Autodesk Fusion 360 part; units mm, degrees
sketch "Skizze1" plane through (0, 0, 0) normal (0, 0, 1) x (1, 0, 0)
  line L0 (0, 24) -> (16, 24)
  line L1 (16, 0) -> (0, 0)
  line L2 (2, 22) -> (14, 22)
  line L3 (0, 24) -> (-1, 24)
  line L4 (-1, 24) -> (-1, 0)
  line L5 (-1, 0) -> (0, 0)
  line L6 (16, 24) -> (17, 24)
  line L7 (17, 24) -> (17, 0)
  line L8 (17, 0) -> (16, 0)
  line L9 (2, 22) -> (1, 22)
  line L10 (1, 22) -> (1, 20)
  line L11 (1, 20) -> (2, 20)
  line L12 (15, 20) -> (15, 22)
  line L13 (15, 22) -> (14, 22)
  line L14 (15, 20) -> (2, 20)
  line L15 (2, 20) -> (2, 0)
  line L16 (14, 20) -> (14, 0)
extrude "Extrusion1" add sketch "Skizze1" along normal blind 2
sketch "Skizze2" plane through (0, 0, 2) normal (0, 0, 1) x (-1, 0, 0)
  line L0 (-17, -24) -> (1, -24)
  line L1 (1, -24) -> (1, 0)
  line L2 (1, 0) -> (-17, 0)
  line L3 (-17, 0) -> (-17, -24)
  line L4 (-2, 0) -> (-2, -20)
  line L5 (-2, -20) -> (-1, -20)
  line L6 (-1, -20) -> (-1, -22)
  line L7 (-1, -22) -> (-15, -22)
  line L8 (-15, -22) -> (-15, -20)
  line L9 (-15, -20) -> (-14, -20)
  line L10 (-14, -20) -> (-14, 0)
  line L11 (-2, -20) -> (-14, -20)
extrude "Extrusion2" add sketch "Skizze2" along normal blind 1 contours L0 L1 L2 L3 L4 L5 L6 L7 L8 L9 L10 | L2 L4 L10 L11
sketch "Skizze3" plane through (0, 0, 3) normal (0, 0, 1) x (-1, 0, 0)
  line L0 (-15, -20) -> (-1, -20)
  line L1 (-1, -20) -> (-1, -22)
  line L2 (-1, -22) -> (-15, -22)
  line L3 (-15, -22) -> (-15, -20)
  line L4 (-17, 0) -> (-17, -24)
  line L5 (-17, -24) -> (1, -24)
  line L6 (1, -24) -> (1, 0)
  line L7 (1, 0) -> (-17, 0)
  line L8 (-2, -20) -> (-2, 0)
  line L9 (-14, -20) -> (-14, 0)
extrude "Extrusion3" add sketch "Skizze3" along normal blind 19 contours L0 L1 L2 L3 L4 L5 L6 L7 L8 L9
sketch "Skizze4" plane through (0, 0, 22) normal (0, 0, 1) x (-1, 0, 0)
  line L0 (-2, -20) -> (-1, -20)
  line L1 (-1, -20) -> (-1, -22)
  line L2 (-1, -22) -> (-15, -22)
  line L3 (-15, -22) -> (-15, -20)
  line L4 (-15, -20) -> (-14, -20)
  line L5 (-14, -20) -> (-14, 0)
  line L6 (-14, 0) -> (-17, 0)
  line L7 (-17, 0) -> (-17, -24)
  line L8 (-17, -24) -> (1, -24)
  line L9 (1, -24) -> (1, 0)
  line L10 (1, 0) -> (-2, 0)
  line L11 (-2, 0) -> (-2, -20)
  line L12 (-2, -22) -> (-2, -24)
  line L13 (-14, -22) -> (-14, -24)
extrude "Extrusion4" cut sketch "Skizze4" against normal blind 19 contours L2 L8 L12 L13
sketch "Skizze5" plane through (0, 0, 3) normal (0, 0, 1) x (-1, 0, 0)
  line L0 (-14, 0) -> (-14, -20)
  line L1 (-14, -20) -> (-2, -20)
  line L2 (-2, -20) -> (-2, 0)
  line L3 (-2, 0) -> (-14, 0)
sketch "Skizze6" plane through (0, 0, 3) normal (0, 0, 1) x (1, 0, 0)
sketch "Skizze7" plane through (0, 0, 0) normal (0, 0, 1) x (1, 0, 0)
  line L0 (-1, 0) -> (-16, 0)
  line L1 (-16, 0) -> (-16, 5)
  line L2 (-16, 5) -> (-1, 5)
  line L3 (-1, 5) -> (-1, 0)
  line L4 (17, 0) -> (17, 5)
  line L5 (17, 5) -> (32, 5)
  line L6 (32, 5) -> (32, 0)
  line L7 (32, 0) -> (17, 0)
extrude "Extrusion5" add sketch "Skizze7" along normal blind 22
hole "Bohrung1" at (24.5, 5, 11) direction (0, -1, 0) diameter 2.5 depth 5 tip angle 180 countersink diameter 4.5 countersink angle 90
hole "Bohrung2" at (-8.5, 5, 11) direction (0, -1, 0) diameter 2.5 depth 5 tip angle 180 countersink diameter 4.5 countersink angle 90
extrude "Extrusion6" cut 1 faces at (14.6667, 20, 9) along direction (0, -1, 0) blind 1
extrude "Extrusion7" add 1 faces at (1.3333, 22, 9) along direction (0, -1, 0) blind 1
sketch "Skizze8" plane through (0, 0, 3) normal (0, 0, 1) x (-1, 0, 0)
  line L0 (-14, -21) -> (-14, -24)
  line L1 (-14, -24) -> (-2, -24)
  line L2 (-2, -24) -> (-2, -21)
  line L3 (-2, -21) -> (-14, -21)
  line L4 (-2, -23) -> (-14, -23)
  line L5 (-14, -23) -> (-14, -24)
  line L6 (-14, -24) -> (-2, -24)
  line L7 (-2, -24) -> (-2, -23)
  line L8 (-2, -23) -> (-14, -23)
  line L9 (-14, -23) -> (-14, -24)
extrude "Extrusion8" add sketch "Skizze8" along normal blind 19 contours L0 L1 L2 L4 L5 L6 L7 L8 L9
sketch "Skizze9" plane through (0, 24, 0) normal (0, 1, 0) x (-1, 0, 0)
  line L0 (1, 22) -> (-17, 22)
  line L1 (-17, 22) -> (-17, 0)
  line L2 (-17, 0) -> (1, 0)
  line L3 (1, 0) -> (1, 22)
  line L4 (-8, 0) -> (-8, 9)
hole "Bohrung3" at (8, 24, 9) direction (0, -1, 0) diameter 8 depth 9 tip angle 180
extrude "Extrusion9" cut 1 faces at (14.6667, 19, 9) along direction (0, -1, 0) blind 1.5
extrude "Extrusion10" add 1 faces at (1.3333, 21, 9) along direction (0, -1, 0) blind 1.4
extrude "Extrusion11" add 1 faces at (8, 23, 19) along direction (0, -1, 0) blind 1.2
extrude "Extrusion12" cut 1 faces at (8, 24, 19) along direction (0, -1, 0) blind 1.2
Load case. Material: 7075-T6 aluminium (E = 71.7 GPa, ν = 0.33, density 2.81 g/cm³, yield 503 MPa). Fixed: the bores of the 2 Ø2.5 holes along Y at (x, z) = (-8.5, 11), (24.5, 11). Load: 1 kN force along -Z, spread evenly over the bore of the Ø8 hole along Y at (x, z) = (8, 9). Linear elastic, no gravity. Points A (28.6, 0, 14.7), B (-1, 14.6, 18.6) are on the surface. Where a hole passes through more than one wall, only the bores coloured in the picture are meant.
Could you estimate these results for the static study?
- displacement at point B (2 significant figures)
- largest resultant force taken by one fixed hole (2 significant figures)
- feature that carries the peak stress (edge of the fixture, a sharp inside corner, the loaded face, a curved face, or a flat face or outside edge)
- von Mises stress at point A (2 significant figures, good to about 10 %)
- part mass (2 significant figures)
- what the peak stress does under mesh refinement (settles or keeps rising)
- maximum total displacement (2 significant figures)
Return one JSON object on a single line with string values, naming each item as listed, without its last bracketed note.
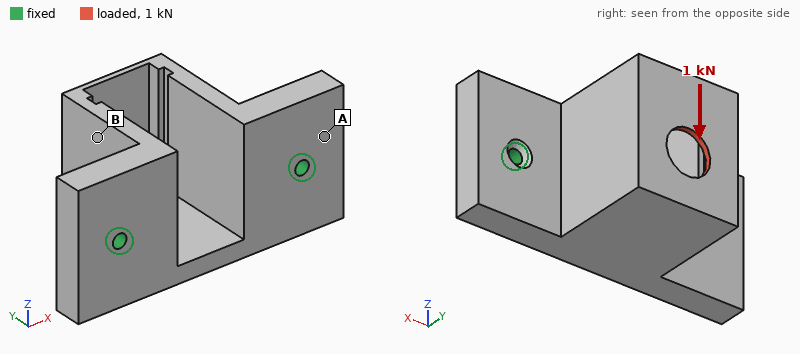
{"displacement at point B": "0.100 mm", "largest resultant force taken by one fixed hole": "620 N", "feature that carries the peak stress": "edge of the fixture", "von Mises stress at point A": "49 MPa", "part mass": "20 g", "what the peak stress does under mesh refinement": "keeps rising", "maximum total displacement": "0.16 mm"}
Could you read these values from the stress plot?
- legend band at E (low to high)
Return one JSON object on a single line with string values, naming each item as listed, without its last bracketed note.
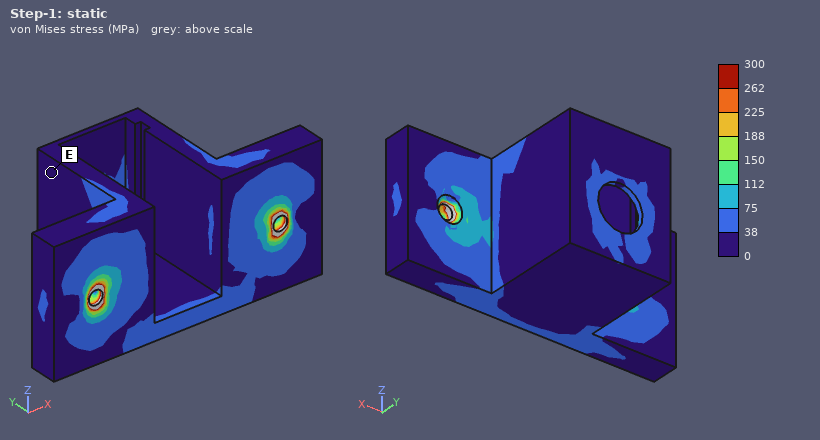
{"legend band at E": "0 to 38 MPa"}
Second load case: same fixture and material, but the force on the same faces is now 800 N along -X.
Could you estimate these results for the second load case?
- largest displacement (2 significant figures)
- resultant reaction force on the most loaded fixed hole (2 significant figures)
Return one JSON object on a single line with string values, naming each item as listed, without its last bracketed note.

{"largest displacement": "0.14 mm", "resultant reaction force on the most loaded fixed hole": "620 N"}
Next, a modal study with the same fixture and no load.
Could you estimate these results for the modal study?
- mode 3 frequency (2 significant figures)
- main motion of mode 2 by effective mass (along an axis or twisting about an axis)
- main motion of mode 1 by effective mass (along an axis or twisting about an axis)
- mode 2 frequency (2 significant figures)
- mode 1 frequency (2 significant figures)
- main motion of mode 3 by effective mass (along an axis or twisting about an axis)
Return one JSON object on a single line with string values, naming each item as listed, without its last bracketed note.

{"mode 3 frequency": "12 kHz", "main motion of mode 2 by effective mass": "along X", "main motion of mode 1 by effective mass": "along Z", "mode 2 frequency": "7100 Hz", "mode 1 frequency": "5900 Hz", "main motion of mode 3 by effective mass": "along Y"}
